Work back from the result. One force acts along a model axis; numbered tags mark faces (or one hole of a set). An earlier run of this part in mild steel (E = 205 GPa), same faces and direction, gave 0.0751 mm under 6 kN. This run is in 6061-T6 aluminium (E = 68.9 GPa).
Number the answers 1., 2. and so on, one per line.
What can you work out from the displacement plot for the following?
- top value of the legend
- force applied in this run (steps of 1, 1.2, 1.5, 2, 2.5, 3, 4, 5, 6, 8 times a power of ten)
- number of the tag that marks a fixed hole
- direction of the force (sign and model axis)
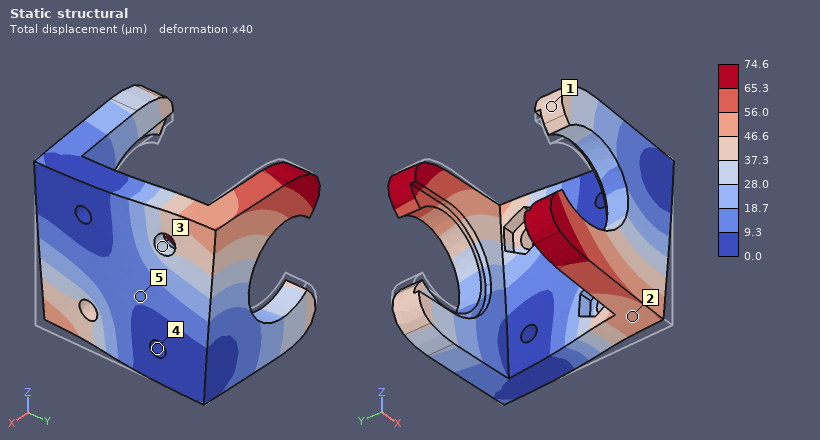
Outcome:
1. 74.6 µm
2. 2 kN
3. 4
4. -X
